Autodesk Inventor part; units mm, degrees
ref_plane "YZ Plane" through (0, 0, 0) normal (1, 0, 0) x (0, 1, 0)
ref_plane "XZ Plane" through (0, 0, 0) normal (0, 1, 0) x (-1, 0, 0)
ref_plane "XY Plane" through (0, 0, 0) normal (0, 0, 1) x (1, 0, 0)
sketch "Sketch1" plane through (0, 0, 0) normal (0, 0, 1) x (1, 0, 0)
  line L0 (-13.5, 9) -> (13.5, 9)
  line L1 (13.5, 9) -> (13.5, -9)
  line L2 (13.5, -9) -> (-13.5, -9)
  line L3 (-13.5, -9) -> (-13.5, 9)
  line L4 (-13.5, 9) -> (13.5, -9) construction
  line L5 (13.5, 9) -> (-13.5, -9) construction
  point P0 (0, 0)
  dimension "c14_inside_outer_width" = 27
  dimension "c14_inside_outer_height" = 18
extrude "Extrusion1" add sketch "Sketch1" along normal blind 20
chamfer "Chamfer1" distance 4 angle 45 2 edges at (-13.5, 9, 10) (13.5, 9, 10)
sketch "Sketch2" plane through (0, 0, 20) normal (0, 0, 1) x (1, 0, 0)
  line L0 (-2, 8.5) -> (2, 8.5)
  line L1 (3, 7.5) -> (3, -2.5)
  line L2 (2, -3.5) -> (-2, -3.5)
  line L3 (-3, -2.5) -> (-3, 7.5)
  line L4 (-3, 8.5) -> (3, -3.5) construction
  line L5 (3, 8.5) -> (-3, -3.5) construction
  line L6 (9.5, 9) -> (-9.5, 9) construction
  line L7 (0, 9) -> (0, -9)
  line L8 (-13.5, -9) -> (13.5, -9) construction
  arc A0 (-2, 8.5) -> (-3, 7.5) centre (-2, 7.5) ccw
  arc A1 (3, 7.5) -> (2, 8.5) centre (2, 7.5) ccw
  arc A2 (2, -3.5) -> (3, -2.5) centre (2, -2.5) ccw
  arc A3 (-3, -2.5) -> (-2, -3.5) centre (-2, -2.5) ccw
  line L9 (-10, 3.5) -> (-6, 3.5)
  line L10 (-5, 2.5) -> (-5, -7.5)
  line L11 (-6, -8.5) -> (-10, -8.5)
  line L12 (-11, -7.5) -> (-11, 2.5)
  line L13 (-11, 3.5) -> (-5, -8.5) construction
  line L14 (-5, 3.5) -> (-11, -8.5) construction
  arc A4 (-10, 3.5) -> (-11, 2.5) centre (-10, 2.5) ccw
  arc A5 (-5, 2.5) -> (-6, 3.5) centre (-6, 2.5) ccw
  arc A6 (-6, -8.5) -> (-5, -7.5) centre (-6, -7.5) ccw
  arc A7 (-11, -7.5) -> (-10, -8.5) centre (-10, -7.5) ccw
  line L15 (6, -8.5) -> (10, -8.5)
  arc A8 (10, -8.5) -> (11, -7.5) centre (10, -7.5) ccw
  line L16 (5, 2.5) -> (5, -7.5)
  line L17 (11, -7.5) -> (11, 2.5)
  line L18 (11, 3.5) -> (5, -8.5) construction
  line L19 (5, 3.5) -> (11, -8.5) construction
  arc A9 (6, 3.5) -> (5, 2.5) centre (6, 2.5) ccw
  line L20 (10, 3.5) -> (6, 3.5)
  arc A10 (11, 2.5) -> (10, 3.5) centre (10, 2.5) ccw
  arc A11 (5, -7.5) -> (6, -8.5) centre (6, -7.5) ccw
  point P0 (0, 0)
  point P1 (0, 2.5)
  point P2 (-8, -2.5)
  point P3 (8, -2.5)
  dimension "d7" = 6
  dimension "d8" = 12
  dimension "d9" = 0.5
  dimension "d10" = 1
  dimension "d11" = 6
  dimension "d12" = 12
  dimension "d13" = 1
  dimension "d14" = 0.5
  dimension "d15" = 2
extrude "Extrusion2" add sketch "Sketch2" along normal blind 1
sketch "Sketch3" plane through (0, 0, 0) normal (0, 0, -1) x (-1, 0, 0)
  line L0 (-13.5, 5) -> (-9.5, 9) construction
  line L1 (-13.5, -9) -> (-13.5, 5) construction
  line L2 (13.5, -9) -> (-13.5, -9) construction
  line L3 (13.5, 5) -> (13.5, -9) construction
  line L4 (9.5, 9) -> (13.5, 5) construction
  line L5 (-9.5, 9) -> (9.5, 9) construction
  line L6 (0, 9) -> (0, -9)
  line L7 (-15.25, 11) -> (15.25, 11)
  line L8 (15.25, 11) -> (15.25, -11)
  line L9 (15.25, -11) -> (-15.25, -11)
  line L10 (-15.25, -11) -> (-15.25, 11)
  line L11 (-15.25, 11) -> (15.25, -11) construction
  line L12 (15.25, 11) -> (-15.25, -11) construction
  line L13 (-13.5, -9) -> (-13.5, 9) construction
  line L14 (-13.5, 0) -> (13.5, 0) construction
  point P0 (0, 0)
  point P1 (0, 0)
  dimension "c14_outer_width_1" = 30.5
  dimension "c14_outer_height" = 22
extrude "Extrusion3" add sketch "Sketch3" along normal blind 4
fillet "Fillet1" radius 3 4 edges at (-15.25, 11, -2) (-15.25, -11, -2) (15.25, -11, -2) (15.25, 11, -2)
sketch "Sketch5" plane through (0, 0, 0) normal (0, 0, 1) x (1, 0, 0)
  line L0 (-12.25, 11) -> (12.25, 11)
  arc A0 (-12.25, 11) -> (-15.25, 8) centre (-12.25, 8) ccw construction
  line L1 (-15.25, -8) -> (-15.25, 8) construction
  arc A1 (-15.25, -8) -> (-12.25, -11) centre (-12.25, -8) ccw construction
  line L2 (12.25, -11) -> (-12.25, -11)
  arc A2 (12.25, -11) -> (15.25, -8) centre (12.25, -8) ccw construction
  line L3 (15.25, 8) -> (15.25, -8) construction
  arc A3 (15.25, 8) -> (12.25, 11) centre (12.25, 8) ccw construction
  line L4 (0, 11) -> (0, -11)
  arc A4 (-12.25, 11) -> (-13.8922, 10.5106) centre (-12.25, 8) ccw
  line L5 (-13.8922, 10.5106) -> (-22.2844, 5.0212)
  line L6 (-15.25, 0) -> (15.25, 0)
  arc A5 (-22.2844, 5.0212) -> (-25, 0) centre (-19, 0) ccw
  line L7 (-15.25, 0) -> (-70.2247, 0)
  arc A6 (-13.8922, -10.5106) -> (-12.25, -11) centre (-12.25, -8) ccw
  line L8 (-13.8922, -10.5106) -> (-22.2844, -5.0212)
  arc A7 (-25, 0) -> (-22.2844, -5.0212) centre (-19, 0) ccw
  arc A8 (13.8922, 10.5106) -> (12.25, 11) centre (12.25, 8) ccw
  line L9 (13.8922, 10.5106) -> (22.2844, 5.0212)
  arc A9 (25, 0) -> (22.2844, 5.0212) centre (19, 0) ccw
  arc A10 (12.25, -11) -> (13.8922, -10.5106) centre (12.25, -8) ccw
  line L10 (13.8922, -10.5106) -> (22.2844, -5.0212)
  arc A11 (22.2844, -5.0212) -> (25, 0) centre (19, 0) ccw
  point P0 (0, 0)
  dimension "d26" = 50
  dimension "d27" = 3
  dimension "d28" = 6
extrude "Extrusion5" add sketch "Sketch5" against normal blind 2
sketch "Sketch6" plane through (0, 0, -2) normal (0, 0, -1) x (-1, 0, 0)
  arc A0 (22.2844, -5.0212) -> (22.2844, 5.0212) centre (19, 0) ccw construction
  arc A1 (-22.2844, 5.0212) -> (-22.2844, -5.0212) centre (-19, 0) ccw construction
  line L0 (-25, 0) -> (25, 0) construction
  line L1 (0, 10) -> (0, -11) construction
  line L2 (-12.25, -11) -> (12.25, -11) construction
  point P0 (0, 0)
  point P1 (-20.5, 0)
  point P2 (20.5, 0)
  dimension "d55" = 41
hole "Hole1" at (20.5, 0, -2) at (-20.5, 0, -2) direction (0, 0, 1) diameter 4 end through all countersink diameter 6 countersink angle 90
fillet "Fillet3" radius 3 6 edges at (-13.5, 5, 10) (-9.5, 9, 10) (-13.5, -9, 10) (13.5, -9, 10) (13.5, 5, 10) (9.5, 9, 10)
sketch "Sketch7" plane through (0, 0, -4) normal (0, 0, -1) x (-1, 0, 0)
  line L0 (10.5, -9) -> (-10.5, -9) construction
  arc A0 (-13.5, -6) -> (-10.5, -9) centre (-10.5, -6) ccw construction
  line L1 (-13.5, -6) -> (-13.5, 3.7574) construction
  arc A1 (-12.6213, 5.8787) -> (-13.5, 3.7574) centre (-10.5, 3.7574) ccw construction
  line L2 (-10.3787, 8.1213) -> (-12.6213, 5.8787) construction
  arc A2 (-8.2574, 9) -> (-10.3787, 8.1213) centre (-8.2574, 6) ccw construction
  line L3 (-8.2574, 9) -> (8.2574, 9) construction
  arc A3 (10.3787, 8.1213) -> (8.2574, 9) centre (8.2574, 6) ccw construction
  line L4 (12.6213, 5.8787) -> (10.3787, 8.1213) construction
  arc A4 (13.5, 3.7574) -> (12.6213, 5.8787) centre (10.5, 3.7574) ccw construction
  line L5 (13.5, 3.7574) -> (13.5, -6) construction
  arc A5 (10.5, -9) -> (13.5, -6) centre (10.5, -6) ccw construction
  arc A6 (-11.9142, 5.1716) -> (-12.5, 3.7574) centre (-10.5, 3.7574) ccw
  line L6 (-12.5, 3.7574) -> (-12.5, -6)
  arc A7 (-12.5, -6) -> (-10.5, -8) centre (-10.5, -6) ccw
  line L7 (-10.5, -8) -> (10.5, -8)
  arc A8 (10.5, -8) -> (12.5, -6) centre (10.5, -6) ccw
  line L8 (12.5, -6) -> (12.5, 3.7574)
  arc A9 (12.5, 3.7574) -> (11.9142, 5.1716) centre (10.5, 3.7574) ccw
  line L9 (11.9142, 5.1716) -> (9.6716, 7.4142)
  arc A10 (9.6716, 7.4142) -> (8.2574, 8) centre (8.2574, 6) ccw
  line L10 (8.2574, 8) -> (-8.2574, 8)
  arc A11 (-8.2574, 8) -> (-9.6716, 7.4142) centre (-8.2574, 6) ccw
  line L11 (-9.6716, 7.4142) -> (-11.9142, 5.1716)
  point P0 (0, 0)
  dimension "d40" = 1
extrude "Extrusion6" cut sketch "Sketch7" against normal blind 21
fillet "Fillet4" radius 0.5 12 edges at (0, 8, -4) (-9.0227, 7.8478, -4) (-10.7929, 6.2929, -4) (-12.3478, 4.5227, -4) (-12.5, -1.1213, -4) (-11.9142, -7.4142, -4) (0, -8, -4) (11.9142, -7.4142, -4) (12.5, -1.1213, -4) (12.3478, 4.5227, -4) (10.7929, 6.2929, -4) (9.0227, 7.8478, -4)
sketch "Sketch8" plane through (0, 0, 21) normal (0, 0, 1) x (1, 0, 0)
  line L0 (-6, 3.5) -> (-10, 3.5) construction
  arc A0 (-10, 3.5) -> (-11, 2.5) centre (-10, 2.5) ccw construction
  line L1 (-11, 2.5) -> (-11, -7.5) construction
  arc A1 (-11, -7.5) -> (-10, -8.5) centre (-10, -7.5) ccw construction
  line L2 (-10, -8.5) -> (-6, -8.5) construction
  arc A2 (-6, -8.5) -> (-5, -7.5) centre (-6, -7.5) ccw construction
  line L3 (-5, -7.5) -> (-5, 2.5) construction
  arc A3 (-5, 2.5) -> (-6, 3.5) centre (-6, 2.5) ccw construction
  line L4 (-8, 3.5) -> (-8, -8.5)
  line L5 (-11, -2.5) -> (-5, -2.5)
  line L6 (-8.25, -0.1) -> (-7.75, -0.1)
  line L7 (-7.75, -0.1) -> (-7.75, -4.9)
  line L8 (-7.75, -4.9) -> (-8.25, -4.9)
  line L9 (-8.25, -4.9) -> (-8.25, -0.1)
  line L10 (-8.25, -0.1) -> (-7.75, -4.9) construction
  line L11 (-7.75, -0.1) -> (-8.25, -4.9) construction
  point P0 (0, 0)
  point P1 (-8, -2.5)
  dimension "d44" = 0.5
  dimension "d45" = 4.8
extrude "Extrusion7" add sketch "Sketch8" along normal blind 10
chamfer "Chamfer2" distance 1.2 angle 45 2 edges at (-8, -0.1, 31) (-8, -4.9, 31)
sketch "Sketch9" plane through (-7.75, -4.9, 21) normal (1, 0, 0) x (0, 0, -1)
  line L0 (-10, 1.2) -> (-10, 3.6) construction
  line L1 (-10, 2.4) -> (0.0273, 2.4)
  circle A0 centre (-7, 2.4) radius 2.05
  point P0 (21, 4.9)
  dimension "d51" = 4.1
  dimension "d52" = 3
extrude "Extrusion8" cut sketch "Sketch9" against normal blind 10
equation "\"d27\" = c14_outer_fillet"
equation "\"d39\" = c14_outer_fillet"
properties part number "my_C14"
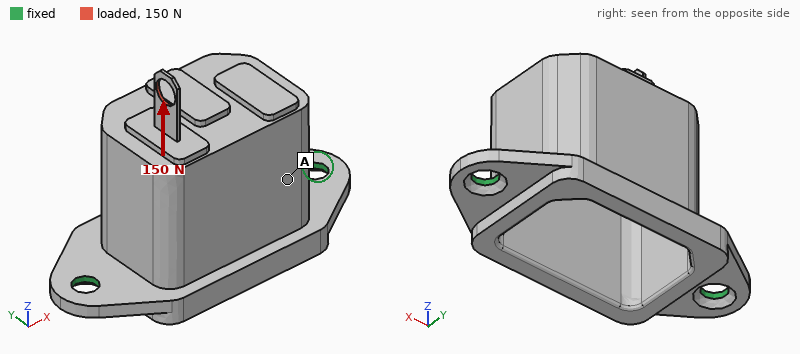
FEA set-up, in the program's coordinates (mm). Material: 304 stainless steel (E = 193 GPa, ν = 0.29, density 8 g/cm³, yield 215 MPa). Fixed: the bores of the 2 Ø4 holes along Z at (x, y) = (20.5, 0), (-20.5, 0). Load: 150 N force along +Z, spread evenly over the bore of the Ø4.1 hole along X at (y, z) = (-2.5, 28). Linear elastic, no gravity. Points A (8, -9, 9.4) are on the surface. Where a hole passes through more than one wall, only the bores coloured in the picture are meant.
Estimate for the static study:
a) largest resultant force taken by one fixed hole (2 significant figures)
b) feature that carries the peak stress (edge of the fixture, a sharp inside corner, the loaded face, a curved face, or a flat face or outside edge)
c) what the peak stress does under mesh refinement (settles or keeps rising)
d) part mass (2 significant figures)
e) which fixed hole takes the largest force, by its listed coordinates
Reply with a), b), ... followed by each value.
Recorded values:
a) 110 N
b) a sharp inside corner
c) keeps rising
d) 36 g
e) (-20.5, 0)
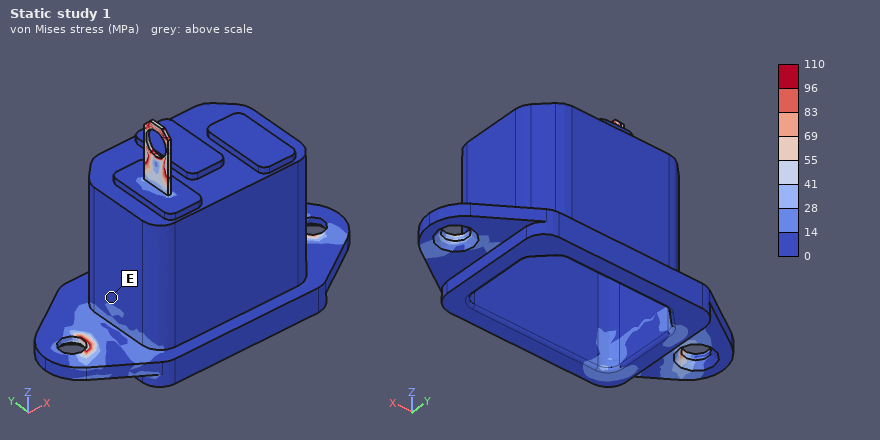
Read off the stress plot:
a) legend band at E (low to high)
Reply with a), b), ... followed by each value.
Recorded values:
a) 0 to 14 MPa
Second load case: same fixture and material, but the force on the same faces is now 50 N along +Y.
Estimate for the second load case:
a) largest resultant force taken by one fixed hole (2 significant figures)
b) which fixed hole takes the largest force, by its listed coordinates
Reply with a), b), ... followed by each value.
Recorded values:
a) 32 N
b) (-20.5, 0)
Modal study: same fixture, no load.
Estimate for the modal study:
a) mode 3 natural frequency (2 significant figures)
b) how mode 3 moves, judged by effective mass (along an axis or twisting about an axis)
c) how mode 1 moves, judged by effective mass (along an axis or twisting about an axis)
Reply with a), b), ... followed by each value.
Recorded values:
a) 5900 Hz
b) along X
c) along Y
